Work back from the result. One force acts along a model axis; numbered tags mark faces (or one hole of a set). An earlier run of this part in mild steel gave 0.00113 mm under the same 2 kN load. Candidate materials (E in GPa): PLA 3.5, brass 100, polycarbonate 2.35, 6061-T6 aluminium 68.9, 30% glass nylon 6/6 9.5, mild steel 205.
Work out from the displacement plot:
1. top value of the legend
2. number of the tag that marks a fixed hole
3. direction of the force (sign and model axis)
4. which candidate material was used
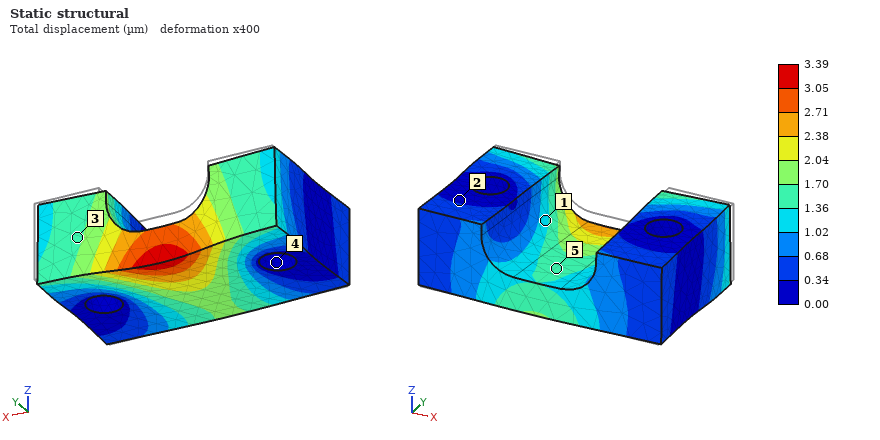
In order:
3.39 µm
4
-Y
6061-T6 aluminium
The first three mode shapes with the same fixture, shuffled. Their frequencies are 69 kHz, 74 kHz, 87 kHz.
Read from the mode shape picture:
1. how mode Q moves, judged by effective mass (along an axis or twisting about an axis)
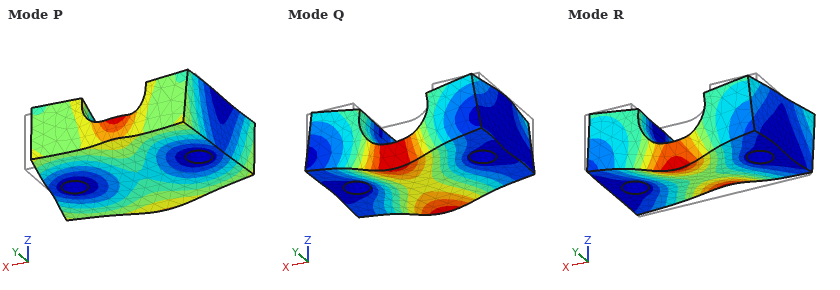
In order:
along Z
